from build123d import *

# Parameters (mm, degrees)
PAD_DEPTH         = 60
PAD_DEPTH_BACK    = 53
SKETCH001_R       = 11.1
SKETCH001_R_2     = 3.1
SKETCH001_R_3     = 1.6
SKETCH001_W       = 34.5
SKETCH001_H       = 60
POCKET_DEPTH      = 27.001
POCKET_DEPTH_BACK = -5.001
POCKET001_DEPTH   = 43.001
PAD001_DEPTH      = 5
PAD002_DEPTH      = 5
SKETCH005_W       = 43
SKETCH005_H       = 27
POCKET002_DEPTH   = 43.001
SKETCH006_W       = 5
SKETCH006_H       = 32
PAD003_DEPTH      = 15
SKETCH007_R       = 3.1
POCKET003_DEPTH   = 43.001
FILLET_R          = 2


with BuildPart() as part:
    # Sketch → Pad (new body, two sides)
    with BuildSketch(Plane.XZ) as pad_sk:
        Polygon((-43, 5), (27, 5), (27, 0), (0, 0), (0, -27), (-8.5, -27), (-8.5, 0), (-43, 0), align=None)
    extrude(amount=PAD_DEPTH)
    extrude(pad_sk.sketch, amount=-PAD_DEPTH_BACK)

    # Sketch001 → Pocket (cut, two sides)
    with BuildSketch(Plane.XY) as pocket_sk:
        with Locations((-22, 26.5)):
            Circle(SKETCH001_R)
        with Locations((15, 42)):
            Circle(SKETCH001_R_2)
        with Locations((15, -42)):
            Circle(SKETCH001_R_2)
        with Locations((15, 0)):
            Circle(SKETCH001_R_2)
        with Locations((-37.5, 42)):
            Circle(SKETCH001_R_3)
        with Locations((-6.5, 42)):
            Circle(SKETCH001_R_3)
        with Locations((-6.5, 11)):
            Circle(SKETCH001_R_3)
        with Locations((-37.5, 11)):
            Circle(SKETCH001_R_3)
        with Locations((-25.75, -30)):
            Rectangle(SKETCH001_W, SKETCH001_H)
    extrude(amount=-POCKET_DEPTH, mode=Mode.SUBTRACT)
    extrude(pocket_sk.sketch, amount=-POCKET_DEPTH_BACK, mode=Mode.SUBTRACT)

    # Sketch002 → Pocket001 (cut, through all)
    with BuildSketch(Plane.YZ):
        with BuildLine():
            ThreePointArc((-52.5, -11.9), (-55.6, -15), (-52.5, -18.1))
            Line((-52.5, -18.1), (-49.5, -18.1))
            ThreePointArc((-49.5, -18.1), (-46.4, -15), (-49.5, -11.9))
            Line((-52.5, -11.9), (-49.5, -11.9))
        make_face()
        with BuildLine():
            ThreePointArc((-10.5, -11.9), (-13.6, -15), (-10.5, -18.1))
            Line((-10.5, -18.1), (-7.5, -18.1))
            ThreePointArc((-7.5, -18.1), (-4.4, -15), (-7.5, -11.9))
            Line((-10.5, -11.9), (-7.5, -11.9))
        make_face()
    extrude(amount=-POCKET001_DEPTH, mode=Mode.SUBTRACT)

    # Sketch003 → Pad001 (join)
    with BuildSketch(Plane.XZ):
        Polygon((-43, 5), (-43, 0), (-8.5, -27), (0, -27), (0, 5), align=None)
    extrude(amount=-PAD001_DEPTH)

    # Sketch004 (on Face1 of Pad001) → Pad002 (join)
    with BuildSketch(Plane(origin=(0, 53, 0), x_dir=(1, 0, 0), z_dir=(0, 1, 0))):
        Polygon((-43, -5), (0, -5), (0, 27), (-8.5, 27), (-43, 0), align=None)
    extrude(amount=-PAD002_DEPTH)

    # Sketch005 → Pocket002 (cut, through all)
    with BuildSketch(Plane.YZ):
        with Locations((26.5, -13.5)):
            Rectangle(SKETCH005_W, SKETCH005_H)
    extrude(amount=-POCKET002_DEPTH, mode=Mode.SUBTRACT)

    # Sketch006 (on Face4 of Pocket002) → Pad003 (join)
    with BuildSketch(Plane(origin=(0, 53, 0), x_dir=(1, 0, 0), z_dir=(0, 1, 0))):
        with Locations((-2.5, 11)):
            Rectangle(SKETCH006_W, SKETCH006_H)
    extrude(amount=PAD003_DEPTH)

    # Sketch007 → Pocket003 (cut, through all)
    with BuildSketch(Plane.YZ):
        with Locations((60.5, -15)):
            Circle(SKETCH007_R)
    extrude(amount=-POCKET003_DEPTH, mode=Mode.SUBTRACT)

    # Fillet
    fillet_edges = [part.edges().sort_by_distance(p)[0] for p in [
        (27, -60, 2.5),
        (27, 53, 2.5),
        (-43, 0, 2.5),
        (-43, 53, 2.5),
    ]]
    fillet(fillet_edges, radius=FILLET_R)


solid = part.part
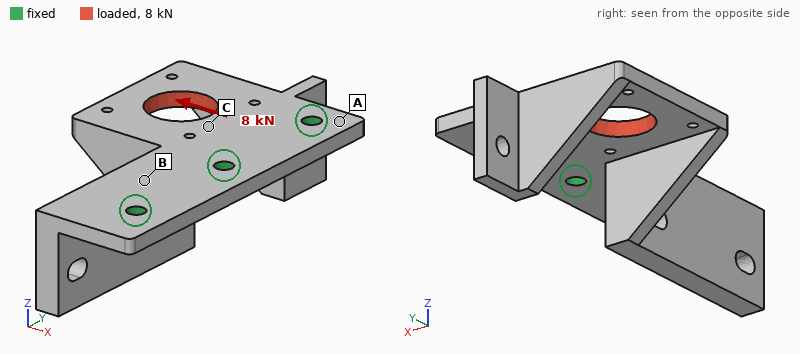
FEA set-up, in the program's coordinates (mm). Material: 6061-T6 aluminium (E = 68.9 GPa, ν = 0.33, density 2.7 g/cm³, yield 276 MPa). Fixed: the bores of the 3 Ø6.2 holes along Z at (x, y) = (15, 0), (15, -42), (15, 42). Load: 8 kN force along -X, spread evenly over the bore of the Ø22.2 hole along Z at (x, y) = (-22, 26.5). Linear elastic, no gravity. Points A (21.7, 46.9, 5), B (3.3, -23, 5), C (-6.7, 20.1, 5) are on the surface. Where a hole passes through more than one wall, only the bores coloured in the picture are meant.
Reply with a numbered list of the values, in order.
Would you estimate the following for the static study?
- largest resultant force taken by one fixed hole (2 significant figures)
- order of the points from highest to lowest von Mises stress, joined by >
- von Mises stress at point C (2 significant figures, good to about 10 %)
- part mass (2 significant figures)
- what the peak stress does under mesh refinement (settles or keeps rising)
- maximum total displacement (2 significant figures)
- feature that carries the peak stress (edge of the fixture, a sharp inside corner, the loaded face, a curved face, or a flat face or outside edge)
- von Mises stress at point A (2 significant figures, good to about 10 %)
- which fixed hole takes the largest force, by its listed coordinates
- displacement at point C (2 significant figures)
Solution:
1. 5.1 kN
2. C > A > B
3. 30 MPa
4. 130 g
5. keeps rising
6. 44 µm
7. edge of the fixture
8. 20 MPa
9. (15, 42)
10. 13 µm
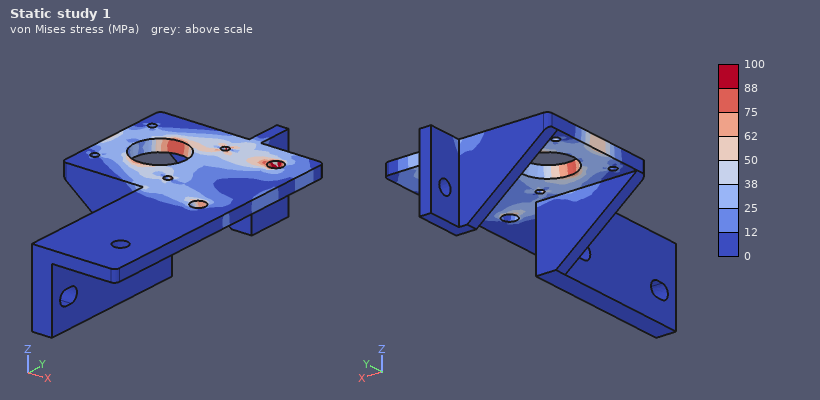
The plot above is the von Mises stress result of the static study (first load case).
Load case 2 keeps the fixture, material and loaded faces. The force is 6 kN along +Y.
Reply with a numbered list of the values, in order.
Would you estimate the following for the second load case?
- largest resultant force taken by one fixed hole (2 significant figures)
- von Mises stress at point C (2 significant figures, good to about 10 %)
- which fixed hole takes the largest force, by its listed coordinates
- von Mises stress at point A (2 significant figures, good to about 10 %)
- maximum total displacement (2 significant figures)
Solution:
1. 4.4 kN
2. 67 MPa
3. (15, 42)
4. 24 MPa
5. 98 µm
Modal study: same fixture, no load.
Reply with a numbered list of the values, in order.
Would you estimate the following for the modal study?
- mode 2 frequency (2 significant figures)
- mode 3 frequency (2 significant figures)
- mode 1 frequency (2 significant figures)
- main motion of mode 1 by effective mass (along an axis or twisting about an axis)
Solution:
1. 1900 Hz
2. 2900 Hz
3. 1300 Hz
4. along Z
